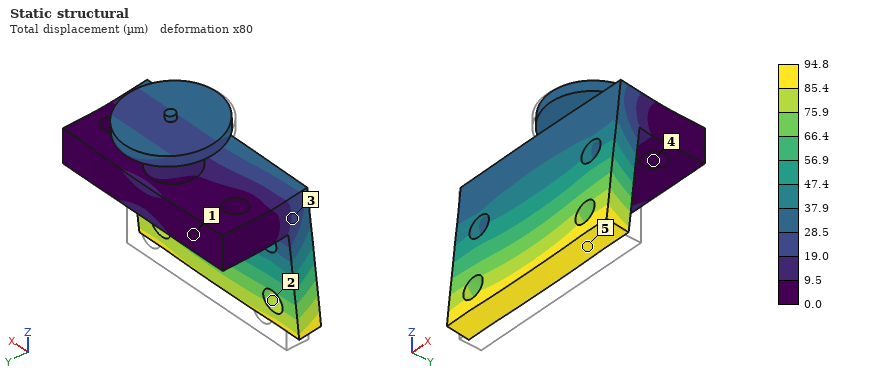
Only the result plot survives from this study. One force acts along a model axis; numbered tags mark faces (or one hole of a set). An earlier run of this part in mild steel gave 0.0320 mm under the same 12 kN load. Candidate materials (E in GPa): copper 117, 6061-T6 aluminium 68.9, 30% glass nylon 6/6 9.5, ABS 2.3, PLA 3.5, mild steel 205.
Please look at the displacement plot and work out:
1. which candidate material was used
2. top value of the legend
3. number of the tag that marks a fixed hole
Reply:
6061-T6 aluminium
94.8 µm
4
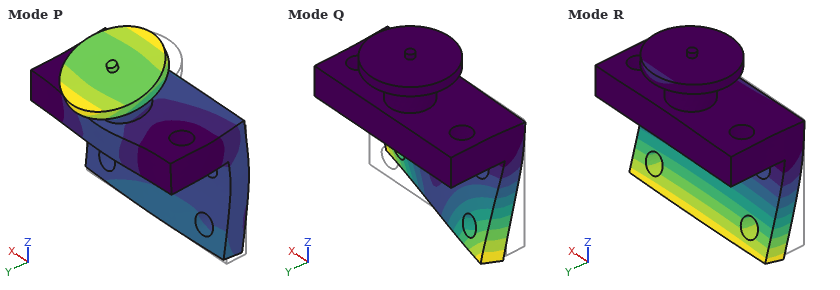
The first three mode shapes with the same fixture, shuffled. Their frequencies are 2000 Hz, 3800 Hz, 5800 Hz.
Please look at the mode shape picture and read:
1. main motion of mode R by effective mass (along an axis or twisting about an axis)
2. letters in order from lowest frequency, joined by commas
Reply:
along Y
R, Q, P
